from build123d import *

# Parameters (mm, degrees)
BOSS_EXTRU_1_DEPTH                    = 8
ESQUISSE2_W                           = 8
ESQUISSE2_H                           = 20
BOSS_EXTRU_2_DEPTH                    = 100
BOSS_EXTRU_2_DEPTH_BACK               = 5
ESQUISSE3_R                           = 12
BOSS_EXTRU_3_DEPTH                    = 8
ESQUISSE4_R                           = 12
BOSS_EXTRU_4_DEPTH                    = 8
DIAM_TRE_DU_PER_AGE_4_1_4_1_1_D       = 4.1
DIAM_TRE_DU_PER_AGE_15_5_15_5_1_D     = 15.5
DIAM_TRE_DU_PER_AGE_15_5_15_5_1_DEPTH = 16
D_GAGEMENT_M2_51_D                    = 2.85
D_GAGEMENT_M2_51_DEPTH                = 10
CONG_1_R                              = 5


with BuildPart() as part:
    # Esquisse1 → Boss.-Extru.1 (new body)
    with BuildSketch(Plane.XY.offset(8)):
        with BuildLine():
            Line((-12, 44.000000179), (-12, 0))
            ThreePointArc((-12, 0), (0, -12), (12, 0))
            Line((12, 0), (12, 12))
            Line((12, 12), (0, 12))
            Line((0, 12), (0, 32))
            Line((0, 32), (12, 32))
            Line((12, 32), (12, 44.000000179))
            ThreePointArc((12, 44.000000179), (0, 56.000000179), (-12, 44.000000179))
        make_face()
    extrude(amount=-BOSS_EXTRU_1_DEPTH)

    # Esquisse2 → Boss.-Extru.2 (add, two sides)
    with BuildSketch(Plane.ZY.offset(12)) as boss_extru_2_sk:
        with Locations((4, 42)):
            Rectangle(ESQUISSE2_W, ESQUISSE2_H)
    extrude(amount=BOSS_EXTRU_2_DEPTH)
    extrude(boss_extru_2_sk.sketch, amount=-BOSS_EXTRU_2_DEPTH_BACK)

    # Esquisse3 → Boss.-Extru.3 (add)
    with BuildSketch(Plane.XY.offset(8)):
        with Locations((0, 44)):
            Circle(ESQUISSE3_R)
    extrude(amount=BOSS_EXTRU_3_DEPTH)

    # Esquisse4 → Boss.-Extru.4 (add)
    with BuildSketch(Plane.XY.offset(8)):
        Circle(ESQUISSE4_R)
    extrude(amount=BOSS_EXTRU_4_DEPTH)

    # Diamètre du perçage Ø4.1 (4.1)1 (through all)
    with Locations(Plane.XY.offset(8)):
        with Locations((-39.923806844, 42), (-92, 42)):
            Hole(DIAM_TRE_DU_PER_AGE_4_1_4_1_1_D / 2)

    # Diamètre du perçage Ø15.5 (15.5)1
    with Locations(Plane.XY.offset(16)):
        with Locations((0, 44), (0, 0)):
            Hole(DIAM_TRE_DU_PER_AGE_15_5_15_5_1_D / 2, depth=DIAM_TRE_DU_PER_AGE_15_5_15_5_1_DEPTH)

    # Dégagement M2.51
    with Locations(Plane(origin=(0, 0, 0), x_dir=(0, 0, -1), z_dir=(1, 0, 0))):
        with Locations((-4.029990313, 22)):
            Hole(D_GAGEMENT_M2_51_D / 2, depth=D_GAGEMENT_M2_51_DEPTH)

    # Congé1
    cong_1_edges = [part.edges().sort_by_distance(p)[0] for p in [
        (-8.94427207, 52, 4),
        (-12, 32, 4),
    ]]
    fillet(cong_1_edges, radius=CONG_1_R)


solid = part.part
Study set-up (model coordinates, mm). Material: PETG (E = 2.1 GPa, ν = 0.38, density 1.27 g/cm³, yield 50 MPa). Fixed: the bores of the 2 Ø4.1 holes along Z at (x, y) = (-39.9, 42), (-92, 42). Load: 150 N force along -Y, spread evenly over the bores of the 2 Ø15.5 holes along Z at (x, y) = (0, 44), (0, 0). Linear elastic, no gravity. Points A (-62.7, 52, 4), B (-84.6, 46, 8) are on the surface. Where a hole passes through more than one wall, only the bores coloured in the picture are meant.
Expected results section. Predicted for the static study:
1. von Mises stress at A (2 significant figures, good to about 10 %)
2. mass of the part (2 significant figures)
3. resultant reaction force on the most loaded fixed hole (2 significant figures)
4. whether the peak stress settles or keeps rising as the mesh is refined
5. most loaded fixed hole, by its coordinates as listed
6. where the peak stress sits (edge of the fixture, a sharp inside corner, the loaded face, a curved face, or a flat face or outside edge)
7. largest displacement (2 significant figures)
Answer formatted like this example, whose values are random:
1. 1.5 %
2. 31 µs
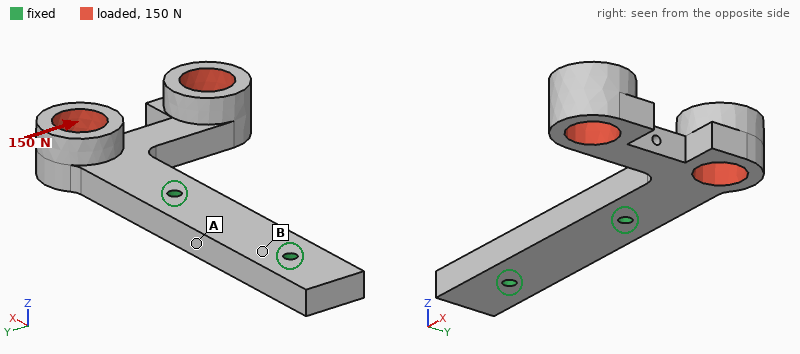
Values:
1. 3.5 MPa
2. 35 g
3. 230 N
4. keeps rising
5. (-39.9, 42)
6. edge of the fixture
7. 1.7 mm
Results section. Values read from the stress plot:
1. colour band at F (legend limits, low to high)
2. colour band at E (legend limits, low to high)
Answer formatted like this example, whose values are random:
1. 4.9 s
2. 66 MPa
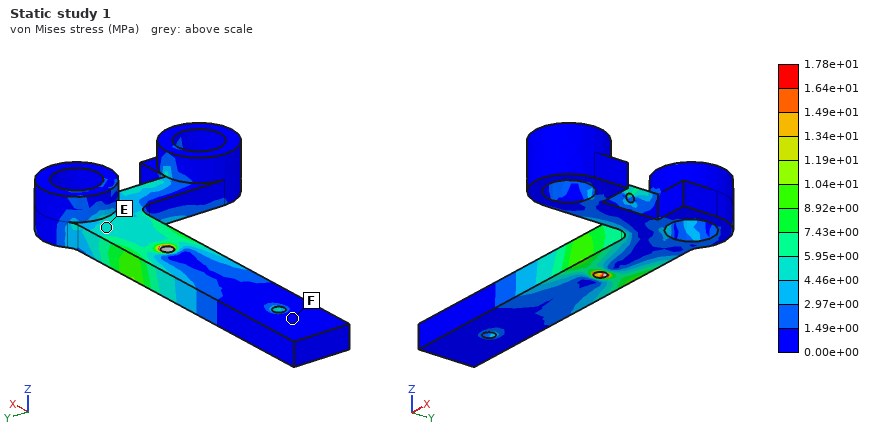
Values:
1. 0.00e+00 to 1.49e+00 MPa
2. 4.46e+00 to 5.95e+00 MPa
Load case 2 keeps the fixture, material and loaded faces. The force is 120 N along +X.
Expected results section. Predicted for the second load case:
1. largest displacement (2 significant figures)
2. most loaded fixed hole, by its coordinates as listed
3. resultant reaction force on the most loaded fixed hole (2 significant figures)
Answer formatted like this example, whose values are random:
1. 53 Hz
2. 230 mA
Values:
1. 1.6 mm
2. (-39.9, 42)
3. 120 N
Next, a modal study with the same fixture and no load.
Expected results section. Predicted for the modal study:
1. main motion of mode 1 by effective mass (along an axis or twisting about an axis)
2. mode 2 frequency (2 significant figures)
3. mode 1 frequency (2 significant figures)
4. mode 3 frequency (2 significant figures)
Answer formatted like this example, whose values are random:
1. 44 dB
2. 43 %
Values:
1. along Z
2. 410 Hz
3. 250 Hz
4. 560 Hz
